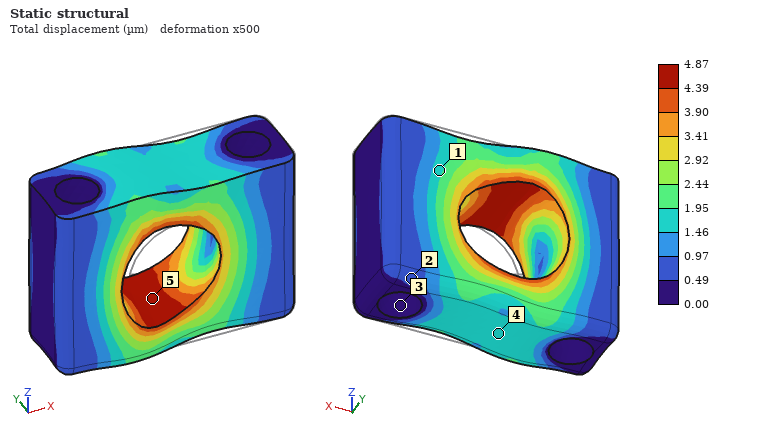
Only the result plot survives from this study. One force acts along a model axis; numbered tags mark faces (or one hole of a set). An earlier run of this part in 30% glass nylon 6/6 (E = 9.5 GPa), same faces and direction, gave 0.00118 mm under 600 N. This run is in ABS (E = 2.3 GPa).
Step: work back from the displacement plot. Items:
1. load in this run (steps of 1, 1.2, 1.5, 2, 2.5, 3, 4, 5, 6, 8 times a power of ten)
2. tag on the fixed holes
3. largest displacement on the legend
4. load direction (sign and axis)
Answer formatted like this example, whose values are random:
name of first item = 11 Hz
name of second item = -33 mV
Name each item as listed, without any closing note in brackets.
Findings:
load in this run = 600 N
tag on the fixed holes = 3
largest displacement on the legend = 4.87 µm
load direction = -X
